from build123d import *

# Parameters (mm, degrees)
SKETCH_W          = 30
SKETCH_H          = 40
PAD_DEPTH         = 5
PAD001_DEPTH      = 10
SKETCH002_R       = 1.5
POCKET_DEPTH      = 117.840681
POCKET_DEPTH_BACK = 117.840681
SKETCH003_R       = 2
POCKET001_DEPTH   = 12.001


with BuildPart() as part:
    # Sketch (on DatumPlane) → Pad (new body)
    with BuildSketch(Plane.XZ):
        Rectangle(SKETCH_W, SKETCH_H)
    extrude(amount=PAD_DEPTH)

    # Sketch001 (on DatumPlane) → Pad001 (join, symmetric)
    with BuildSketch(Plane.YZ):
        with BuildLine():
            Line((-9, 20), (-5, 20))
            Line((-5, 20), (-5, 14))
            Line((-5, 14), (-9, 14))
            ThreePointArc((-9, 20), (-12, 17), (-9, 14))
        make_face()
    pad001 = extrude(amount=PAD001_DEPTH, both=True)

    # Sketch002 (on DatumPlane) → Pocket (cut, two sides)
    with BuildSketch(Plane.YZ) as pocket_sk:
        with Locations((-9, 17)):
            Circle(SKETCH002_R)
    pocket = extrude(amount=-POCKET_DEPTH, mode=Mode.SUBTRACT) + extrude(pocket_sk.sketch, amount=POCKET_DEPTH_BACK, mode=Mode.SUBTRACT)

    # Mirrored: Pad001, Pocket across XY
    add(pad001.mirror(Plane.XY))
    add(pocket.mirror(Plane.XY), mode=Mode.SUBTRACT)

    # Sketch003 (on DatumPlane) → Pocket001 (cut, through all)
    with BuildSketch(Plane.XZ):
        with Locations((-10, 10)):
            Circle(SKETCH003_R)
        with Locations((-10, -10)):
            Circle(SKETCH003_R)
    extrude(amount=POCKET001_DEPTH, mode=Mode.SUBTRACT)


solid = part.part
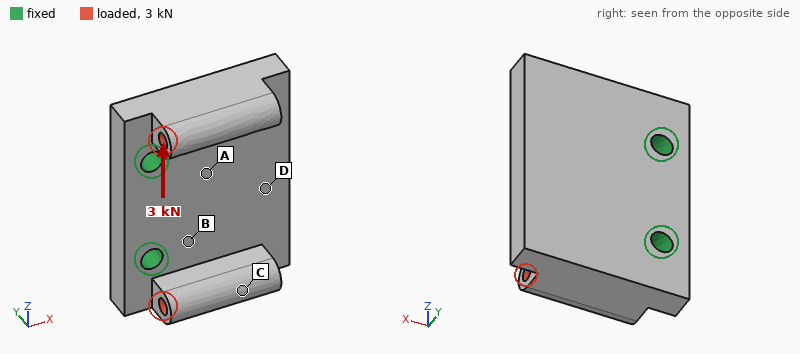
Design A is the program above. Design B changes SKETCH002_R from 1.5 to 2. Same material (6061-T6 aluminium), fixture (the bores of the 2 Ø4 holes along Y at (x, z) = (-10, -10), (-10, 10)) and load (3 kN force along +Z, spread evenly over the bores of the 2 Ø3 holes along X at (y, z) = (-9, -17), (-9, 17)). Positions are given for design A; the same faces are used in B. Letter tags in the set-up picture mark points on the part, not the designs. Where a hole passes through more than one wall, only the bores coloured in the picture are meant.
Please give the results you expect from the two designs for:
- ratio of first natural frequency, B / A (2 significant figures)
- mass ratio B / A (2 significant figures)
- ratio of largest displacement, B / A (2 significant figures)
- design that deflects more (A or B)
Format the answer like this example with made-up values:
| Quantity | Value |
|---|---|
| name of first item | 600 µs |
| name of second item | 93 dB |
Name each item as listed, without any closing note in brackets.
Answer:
| Quantity | Value |
|---|---|
| ratio of first natural frequency, B / A | 1.0 |
| mass ratio B / A | 0.97 |
| ratio of largest displacement, B / A | 1.1 |
| design that deflects more | B |
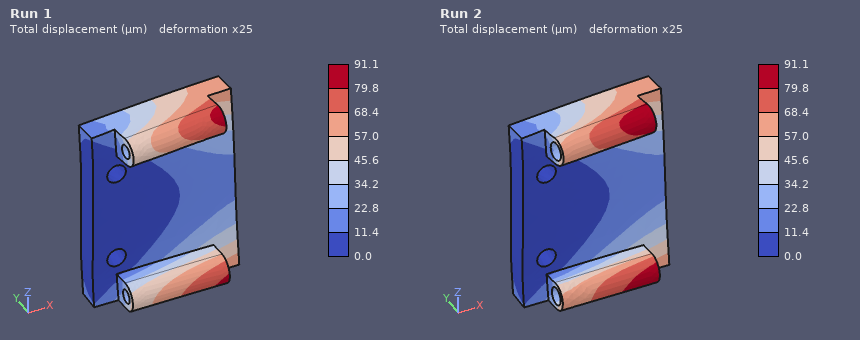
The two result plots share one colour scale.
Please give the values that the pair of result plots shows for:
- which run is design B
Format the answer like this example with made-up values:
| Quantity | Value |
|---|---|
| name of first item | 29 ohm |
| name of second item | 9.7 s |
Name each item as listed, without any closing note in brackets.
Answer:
| Quantity | Value |
|---|---|
| which run is design B | Run 2 |
